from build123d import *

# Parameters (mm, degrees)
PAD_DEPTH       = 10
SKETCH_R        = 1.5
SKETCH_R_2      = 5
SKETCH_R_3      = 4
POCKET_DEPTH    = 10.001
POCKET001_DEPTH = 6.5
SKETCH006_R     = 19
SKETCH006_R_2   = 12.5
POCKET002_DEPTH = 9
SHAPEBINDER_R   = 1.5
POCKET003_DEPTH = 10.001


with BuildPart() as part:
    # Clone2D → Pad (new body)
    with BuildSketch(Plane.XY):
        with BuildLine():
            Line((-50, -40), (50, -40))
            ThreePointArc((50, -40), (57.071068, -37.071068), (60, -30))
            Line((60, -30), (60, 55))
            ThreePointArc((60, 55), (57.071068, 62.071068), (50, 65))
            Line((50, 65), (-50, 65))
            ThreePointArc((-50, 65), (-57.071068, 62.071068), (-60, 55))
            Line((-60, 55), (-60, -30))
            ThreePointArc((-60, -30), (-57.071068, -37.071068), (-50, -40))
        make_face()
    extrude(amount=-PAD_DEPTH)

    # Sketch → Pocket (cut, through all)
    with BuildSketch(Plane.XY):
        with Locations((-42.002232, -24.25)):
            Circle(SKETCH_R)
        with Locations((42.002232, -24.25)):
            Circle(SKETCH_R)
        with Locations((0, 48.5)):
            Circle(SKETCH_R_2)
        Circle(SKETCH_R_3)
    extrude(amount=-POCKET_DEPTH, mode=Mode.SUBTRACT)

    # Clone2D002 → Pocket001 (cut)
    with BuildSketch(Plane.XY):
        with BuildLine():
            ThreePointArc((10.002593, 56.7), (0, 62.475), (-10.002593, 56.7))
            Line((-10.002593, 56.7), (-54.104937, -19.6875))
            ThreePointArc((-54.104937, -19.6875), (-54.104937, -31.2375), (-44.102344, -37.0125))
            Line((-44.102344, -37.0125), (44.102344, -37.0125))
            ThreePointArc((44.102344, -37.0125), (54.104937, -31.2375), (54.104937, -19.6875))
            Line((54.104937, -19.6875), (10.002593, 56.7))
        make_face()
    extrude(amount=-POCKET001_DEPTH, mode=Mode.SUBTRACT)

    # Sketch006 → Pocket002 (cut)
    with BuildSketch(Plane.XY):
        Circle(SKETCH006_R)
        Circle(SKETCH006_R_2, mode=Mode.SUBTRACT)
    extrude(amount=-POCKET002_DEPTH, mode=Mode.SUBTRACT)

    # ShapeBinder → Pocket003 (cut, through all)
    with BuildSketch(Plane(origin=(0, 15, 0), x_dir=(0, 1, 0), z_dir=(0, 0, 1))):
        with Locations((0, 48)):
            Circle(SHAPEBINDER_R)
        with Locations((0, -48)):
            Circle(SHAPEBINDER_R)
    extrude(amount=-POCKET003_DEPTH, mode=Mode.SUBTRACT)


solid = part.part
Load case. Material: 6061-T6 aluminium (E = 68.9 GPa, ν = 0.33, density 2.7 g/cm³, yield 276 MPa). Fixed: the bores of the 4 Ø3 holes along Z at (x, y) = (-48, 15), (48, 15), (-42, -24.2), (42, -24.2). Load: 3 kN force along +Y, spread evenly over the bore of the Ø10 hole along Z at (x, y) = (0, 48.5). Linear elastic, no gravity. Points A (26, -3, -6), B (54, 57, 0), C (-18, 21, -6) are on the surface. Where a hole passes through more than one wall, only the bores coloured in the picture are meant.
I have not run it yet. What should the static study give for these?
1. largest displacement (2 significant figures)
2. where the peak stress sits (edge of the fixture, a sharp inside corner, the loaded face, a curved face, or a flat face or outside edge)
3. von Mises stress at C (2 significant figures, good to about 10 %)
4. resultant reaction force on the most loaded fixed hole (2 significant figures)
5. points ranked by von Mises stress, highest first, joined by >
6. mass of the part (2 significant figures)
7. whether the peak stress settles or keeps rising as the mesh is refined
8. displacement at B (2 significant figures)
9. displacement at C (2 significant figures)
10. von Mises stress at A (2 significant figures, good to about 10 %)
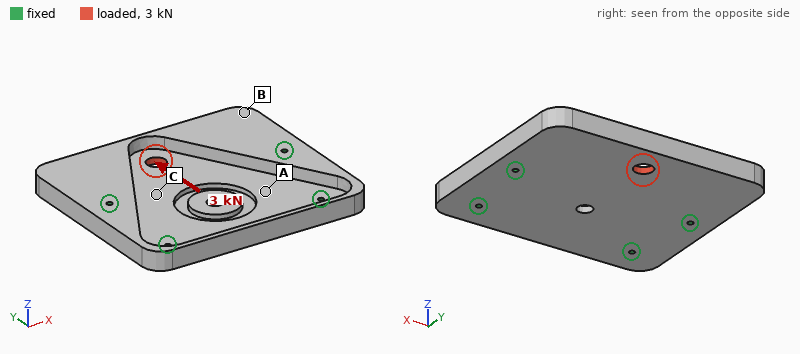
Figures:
32 µm
edge of the fixture
11 MPa
1.2 kN
C > A > B
210 g
keeps rising
14 µm
6.5 µm
7.2 MPa
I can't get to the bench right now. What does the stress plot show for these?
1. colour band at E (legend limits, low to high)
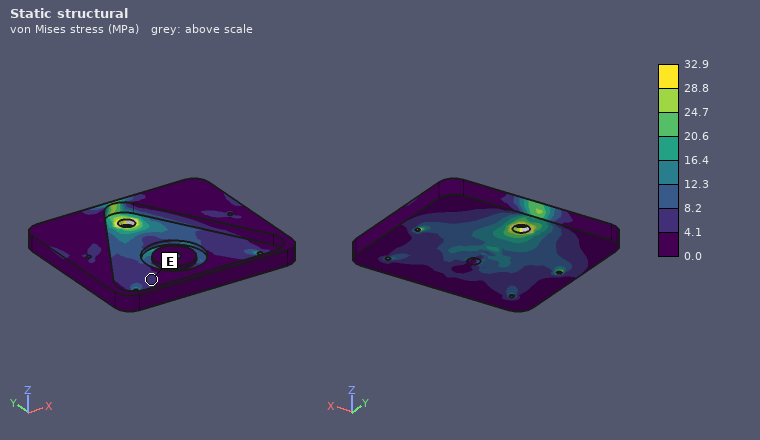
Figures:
4.1 to 8.2 MPa
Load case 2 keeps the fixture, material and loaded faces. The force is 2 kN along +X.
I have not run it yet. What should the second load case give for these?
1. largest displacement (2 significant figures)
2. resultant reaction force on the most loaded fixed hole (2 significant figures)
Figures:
11 µm
1.2 kN
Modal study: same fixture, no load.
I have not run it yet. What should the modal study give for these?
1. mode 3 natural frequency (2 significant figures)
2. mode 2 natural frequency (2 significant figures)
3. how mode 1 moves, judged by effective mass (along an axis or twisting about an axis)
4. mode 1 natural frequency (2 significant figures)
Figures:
3300 Hz
3200 Hz
along Z
2000 Hz
